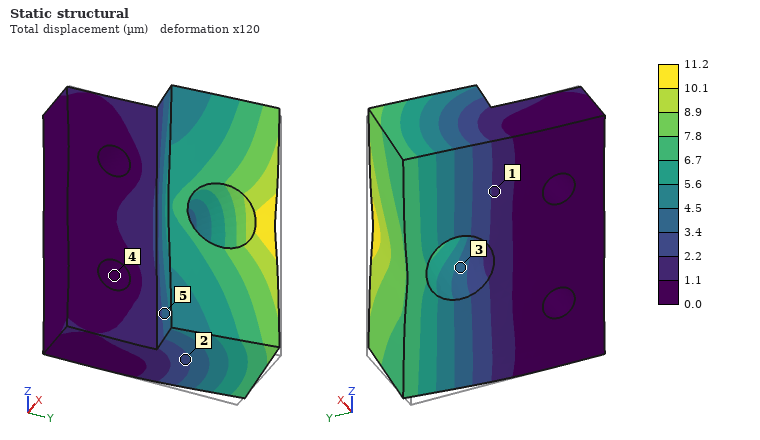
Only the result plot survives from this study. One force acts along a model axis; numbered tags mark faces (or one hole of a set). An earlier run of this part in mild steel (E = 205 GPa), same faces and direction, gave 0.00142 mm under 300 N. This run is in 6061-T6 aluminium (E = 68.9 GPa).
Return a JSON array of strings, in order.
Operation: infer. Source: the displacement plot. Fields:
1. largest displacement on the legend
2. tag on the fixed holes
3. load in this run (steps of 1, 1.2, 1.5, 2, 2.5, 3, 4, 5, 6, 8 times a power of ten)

["11.2 µm", "4", "800 N"]
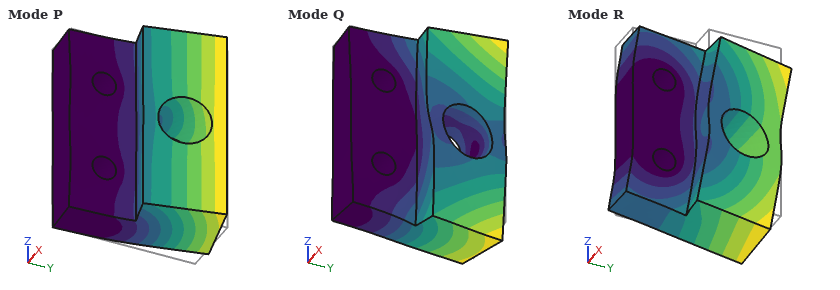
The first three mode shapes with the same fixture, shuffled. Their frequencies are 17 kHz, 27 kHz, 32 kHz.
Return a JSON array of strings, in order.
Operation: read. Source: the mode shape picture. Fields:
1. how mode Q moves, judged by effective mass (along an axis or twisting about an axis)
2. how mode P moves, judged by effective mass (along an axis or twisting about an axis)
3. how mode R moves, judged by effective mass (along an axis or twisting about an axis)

["twisting about Y", "along X", "along Z"]
